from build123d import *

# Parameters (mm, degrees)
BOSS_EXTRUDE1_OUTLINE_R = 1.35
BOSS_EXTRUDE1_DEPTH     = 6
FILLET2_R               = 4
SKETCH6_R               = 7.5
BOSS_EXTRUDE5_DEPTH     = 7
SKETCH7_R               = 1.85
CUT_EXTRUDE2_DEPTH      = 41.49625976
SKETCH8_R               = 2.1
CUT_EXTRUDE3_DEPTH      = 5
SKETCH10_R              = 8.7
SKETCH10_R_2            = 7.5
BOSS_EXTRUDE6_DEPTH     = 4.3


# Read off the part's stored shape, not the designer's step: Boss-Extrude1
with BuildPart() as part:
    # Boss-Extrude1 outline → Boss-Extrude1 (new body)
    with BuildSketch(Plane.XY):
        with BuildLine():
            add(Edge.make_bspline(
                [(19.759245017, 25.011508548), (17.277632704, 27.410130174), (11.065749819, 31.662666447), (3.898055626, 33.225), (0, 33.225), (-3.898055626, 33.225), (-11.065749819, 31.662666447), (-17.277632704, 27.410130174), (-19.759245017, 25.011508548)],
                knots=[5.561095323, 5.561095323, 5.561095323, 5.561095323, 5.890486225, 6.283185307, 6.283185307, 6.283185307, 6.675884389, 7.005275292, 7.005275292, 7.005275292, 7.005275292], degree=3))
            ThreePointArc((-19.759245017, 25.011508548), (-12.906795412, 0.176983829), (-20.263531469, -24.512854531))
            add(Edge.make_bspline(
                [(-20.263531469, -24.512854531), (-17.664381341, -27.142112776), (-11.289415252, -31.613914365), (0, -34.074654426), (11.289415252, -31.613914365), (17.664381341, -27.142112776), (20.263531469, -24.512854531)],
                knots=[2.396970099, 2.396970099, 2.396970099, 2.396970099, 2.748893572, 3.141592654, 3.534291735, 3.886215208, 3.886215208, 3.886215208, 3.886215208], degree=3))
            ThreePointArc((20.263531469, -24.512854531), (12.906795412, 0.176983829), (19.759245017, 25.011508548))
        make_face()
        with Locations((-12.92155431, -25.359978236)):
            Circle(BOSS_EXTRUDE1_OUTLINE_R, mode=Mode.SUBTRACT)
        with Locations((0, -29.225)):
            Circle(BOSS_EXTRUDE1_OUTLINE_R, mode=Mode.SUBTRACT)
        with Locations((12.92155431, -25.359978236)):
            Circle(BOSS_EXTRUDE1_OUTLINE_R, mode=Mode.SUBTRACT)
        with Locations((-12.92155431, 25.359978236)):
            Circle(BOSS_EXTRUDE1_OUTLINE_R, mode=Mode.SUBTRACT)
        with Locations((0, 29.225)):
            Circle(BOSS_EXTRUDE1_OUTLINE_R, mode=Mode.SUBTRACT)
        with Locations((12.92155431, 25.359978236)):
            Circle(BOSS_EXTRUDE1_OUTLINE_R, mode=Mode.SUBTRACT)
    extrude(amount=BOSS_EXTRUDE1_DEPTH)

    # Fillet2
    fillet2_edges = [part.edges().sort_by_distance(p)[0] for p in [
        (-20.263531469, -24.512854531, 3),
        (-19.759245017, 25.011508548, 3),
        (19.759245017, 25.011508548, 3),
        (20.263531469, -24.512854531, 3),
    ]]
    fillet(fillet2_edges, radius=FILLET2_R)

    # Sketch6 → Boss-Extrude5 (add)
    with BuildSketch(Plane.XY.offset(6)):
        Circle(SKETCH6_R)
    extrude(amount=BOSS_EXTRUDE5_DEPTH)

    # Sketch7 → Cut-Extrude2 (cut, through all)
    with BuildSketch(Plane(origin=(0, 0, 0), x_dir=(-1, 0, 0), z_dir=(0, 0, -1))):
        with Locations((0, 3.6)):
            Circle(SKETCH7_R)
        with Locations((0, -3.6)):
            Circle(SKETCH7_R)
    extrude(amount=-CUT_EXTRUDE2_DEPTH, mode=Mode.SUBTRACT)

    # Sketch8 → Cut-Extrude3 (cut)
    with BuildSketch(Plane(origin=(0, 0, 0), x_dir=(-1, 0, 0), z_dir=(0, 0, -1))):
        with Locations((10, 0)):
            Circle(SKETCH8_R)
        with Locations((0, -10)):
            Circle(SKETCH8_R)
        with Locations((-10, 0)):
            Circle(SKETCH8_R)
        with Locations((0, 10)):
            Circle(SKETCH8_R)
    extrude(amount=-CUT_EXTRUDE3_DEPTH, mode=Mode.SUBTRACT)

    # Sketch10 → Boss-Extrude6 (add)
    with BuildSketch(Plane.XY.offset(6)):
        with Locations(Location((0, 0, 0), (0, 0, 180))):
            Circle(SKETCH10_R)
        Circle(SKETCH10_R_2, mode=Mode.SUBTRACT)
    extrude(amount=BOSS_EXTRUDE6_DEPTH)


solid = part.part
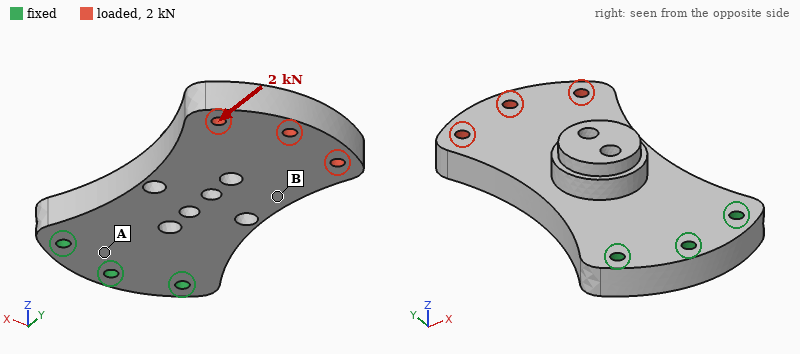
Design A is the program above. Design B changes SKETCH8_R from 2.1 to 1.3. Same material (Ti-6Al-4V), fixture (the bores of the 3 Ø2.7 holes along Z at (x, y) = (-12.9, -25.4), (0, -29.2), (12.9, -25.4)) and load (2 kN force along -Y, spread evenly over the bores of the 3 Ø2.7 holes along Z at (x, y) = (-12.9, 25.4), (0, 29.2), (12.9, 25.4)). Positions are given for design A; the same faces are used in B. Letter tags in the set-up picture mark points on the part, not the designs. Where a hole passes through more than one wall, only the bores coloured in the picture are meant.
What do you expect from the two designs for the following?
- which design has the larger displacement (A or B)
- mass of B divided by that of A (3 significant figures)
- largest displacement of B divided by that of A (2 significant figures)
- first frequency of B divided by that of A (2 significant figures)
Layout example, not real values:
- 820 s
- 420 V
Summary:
- A
- 1.01
- 0.80
- 1.0
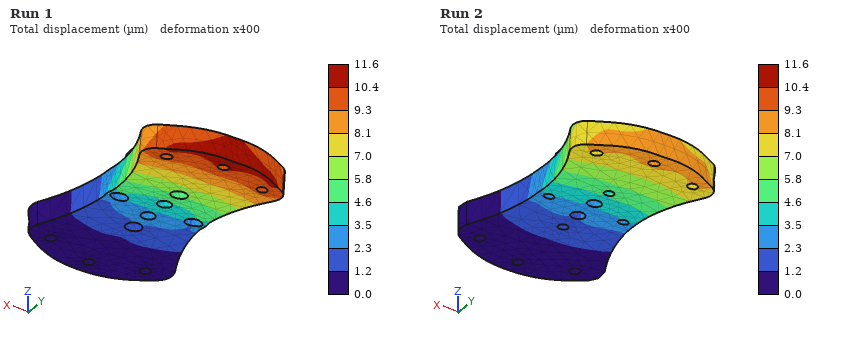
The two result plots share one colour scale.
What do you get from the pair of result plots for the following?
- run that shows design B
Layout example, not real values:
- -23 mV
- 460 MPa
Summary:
- Run 2
